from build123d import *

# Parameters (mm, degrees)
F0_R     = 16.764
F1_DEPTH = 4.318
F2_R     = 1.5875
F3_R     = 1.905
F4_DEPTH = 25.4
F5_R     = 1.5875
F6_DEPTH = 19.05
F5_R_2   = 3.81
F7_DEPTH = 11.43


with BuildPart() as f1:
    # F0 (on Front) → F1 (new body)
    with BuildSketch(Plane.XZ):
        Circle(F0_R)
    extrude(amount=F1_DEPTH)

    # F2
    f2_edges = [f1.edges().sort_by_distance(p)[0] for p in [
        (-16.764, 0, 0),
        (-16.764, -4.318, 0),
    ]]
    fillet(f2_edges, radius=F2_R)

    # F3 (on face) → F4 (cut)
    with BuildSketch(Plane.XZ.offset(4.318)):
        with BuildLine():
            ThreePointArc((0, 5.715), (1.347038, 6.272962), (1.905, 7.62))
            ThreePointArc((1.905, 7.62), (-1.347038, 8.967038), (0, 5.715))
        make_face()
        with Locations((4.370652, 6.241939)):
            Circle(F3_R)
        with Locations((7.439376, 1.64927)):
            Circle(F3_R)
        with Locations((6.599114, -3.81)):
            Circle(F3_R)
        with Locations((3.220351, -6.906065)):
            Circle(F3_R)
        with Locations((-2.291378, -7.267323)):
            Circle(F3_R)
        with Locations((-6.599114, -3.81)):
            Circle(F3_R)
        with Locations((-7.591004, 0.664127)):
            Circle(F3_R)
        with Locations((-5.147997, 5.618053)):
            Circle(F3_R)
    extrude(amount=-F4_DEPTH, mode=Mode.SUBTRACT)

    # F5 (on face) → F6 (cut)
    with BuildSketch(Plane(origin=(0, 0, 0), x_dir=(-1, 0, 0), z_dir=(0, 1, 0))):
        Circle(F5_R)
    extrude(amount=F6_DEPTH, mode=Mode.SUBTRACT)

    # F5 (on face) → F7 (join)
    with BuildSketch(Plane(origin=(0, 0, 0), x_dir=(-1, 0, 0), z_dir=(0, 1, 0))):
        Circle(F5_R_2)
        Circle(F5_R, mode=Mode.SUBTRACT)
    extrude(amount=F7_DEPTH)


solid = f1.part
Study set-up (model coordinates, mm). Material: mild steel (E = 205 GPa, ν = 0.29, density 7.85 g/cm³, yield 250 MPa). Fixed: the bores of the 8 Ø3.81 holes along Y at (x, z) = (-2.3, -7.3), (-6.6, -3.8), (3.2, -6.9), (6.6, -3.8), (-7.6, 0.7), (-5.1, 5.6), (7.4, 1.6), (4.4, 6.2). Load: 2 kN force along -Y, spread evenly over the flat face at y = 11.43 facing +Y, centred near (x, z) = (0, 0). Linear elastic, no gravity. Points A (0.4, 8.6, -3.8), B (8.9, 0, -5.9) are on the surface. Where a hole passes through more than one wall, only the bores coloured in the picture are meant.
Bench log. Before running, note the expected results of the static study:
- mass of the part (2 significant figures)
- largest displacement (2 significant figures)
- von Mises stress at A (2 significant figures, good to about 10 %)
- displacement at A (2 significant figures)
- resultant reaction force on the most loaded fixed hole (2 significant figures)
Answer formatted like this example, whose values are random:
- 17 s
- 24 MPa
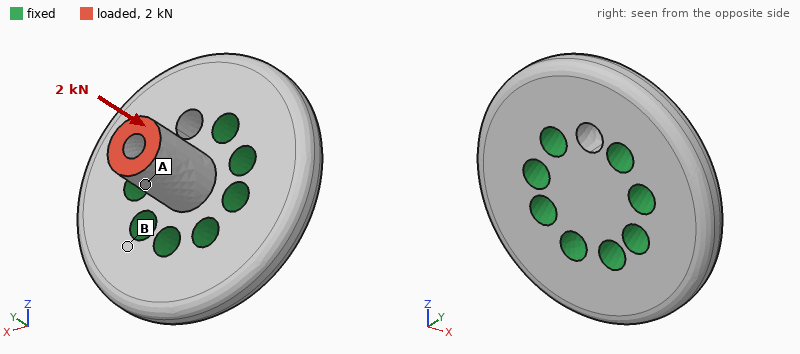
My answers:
- 29 g
- 4.0 µm
- 53 MPa
- 3.1 µm
- 350 N
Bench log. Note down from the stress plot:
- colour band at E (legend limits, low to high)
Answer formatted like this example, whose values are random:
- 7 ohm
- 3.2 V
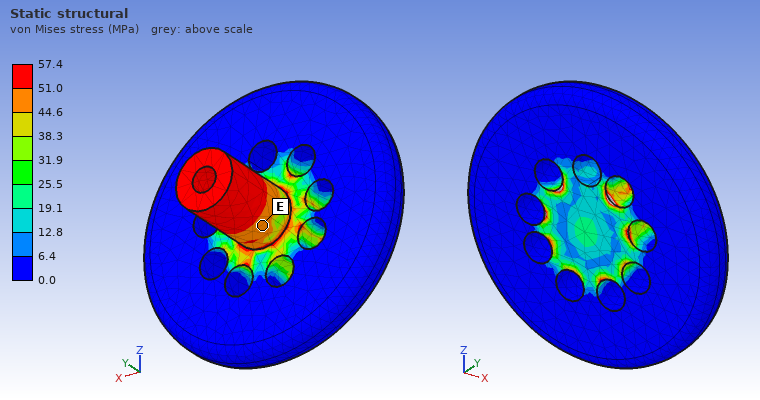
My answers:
- 44.6 to 51.0 MPa
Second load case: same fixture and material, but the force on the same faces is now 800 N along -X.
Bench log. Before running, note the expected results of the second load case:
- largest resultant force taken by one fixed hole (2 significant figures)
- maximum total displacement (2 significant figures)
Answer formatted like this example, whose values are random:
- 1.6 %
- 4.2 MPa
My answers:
- 490 N
- 24 µm
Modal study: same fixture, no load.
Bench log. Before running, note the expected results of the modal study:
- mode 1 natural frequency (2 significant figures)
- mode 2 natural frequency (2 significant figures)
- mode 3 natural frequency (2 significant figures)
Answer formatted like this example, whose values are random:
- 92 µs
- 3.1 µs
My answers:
- 29 kHz
- 29 kHz
- 39 kHz
